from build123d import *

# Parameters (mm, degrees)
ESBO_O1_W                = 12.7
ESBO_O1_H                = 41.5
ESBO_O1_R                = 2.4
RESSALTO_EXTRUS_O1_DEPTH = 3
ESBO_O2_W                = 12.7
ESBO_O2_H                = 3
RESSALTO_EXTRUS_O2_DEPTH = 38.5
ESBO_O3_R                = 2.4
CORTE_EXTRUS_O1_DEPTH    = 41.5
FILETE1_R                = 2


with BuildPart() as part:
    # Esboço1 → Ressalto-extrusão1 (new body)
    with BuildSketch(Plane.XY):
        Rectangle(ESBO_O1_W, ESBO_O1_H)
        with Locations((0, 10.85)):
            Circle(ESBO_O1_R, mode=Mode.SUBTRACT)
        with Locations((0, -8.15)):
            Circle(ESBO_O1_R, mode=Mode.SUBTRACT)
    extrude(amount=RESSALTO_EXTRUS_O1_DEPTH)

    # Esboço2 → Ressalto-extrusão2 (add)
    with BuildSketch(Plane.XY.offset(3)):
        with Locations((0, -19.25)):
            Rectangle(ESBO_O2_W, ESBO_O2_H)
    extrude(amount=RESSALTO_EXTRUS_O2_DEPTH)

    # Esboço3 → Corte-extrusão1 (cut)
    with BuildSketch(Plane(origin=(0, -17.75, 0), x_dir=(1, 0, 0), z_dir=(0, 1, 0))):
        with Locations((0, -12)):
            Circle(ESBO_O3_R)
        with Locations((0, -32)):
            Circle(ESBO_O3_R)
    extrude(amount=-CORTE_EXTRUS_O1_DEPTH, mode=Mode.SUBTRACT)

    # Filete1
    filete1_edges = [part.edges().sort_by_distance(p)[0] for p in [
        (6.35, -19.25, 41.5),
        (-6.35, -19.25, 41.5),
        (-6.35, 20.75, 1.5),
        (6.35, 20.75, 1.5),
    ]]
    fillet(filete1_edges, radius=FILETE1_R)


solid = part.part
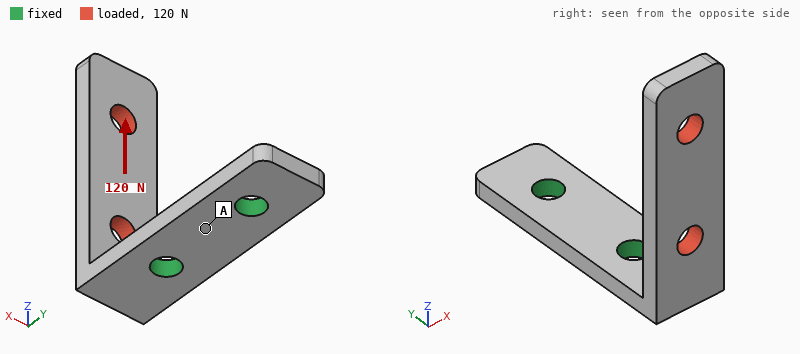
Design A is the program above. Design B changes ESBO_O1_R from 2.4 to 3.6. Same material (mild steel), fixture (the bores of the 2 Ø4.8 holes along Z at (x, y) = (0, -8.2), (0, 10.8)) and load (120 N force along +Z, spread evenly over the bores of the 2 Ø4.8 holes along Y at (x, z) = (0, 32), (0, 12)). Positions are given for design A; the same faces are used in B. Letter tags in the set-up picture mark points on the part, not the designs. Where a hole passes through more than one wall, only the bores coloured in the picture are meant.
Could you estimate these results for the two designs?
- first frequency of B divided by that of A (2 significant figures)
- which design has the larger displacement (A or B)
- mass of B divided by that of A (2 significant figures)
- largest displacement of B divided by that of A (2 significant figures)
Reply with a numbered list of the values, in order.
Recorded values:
1. 1.0
2. A
3. 0.95
4. 0.73
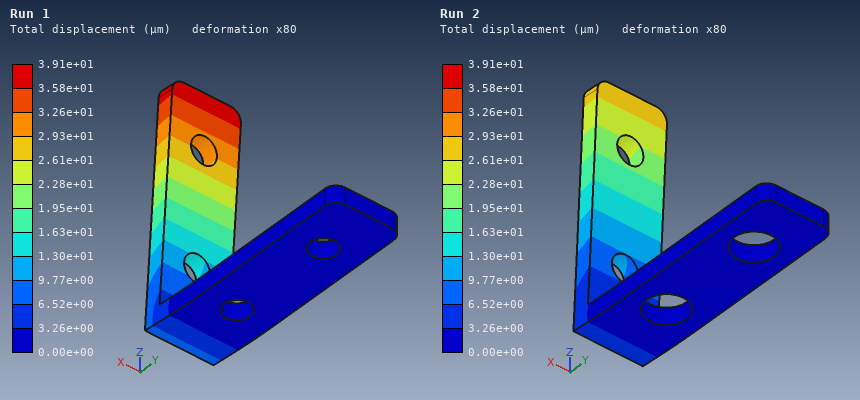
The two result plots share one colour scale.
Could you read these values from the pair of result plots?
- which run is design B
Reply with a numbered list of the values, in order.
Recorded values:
1. Run 2
